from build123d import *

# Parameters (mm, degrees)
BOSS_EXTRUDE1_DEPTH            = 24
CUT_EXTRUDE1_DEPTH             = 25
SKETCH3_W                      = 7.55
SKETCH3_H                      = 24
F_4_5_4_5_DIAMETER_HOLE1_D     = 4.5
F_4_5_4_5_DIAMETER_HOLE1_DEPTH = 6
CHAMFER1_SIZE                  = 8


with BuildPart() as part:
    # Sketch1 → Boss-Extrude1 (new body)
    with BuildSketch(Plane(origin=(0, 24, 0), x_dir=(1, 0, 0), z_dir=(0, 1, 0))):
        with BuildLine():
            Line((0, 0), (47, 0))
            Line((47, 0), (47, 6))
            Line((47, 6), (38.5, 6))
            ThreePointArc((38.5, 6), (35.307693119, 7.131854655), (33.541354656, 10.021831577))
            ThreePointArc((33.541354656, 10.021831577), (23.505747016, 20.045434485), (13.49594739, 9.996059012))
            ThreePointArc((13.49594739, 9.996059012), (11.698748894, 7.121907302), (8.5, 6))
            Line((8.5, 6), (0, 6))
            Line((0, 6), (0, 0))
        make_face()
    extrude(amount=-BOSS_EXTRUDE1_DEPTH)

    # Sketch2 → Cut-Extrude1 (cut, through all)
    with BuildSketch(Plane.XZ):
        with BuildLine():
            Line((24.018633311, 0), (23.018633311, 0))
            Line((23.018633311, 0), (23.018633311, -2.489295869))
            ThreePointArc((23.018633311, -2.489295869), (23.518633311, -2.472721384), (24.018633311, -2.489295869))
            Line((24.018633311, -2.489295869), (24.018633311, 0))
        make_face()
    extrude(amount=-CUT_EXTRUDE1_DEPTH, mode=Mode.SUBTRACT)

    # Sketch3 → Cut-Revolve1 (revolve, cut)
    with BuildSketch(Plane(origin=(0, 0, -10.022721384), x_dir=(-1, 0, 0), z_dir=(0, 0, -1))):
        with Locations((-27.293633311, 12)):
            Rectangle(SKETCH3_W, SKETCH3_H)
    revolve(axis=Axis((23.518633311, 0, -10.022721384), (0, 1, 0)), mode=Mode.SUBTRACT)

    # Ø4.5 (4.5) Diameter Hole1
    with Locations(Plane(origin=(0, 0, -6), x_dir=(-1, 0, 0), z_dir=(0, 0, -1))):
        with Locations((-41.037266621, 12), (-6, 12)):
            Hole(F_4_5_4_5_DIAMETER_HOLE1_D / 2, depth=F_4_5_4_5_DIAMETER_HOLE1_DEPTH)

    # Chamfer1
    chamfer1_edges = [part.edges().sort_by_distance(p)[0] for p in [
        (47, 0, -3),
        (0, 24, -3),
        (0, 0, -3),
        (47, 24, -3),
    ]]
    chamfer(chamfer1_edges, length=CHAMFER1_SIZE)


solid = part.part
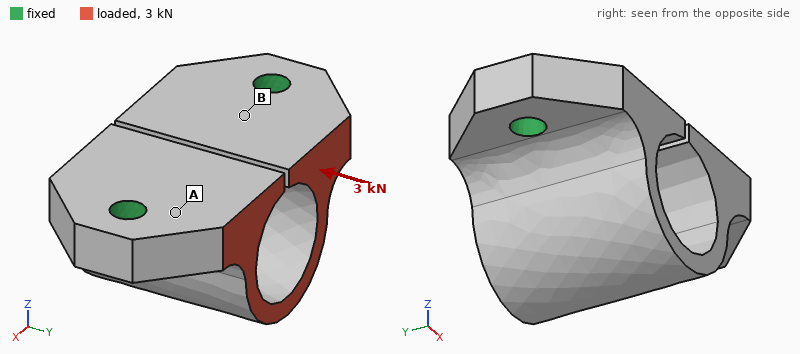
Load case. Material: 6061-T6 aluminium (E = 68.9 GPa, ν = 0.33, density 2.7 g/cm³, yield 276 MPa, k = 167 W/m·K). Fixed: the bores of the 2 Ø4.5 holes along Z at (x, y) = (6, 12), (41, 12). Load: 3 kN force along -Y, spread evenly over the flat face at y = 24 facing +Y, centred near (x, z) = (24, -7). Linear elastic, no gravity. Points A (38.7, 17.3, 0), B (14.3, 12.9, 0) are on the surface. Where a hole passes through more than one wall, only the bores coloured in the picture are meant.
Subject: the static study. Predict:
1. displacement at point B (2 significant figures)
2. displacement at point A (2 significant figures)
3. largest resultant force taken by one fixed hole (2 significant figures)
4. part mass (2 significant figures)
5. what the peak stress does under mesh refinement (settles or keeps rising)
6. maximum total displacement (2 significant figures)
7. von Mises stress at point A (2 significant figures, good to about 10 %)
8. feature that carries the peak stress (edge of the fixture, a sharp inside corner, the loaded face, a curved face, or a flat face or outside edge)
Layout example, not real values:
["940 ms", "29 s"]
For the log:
["9.5 µm", "7.7 µm", "1.5 kN", "20 g", "keeps rising", "50 µm", "27 MPa", "edge of the fixture"]
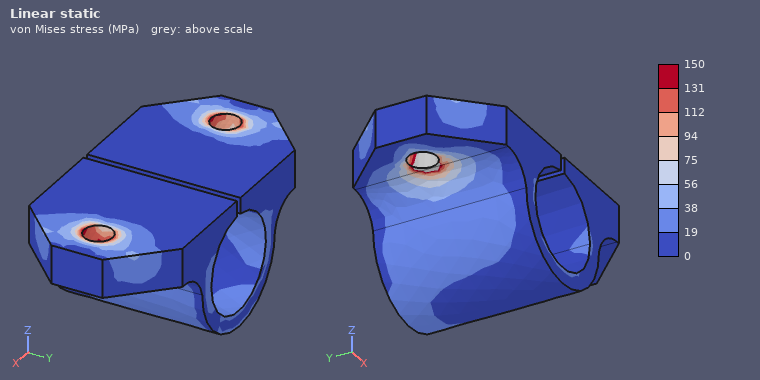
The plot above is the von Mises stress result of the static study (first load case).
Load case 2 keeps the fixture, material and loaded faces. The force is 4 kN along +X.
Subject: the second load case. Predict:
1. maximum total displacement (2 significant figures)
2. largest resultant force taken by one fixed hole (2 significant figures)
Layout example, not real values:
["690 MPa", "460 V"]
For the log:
["72 µm", "2.1 kN"]
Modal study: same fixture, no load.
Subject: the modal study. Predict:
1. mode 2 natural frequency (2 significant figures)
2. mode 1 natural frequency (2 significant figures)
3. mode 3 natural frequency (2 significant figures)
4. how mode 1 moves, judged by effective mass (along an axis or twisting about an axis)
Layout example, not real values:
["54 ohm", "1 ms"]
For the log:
["14 kHz", "11 kHz", "16 kHz", "along Y"]
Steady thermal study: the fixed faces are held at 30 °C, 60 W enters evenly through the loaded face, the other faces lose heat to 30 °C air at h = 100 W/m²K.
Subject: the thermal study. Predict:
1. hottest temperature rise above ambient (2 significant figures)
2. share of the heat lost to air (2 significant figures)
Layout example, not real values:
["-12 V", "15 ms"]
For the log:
["29 K", "7.7 %"]
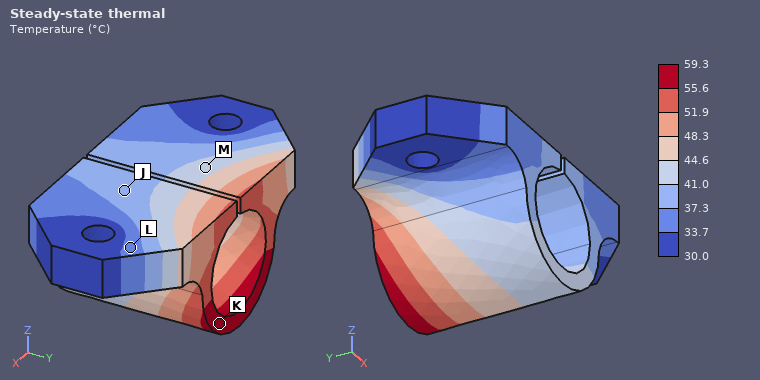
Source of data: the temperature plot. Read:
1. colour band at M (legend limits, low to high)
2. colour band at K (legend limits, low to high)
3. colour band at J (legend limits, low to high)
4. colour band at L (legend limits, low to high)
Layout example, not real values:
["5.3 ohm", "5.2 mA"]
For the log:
["41.0 to 44.6 °C", "55.6 to 59.3 °C", "37.3 to 41.0 °C", "33.7 to 37.3 °C"]
